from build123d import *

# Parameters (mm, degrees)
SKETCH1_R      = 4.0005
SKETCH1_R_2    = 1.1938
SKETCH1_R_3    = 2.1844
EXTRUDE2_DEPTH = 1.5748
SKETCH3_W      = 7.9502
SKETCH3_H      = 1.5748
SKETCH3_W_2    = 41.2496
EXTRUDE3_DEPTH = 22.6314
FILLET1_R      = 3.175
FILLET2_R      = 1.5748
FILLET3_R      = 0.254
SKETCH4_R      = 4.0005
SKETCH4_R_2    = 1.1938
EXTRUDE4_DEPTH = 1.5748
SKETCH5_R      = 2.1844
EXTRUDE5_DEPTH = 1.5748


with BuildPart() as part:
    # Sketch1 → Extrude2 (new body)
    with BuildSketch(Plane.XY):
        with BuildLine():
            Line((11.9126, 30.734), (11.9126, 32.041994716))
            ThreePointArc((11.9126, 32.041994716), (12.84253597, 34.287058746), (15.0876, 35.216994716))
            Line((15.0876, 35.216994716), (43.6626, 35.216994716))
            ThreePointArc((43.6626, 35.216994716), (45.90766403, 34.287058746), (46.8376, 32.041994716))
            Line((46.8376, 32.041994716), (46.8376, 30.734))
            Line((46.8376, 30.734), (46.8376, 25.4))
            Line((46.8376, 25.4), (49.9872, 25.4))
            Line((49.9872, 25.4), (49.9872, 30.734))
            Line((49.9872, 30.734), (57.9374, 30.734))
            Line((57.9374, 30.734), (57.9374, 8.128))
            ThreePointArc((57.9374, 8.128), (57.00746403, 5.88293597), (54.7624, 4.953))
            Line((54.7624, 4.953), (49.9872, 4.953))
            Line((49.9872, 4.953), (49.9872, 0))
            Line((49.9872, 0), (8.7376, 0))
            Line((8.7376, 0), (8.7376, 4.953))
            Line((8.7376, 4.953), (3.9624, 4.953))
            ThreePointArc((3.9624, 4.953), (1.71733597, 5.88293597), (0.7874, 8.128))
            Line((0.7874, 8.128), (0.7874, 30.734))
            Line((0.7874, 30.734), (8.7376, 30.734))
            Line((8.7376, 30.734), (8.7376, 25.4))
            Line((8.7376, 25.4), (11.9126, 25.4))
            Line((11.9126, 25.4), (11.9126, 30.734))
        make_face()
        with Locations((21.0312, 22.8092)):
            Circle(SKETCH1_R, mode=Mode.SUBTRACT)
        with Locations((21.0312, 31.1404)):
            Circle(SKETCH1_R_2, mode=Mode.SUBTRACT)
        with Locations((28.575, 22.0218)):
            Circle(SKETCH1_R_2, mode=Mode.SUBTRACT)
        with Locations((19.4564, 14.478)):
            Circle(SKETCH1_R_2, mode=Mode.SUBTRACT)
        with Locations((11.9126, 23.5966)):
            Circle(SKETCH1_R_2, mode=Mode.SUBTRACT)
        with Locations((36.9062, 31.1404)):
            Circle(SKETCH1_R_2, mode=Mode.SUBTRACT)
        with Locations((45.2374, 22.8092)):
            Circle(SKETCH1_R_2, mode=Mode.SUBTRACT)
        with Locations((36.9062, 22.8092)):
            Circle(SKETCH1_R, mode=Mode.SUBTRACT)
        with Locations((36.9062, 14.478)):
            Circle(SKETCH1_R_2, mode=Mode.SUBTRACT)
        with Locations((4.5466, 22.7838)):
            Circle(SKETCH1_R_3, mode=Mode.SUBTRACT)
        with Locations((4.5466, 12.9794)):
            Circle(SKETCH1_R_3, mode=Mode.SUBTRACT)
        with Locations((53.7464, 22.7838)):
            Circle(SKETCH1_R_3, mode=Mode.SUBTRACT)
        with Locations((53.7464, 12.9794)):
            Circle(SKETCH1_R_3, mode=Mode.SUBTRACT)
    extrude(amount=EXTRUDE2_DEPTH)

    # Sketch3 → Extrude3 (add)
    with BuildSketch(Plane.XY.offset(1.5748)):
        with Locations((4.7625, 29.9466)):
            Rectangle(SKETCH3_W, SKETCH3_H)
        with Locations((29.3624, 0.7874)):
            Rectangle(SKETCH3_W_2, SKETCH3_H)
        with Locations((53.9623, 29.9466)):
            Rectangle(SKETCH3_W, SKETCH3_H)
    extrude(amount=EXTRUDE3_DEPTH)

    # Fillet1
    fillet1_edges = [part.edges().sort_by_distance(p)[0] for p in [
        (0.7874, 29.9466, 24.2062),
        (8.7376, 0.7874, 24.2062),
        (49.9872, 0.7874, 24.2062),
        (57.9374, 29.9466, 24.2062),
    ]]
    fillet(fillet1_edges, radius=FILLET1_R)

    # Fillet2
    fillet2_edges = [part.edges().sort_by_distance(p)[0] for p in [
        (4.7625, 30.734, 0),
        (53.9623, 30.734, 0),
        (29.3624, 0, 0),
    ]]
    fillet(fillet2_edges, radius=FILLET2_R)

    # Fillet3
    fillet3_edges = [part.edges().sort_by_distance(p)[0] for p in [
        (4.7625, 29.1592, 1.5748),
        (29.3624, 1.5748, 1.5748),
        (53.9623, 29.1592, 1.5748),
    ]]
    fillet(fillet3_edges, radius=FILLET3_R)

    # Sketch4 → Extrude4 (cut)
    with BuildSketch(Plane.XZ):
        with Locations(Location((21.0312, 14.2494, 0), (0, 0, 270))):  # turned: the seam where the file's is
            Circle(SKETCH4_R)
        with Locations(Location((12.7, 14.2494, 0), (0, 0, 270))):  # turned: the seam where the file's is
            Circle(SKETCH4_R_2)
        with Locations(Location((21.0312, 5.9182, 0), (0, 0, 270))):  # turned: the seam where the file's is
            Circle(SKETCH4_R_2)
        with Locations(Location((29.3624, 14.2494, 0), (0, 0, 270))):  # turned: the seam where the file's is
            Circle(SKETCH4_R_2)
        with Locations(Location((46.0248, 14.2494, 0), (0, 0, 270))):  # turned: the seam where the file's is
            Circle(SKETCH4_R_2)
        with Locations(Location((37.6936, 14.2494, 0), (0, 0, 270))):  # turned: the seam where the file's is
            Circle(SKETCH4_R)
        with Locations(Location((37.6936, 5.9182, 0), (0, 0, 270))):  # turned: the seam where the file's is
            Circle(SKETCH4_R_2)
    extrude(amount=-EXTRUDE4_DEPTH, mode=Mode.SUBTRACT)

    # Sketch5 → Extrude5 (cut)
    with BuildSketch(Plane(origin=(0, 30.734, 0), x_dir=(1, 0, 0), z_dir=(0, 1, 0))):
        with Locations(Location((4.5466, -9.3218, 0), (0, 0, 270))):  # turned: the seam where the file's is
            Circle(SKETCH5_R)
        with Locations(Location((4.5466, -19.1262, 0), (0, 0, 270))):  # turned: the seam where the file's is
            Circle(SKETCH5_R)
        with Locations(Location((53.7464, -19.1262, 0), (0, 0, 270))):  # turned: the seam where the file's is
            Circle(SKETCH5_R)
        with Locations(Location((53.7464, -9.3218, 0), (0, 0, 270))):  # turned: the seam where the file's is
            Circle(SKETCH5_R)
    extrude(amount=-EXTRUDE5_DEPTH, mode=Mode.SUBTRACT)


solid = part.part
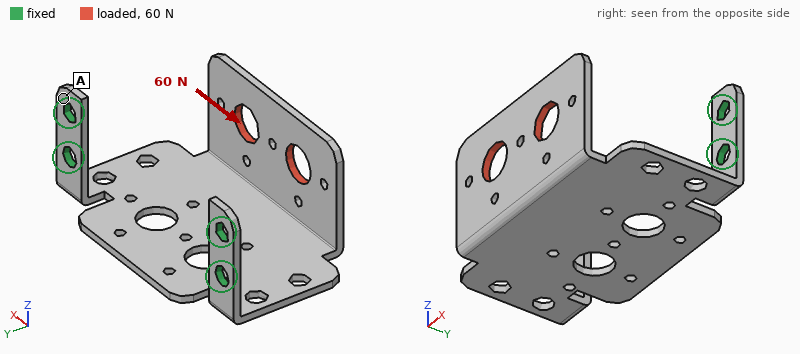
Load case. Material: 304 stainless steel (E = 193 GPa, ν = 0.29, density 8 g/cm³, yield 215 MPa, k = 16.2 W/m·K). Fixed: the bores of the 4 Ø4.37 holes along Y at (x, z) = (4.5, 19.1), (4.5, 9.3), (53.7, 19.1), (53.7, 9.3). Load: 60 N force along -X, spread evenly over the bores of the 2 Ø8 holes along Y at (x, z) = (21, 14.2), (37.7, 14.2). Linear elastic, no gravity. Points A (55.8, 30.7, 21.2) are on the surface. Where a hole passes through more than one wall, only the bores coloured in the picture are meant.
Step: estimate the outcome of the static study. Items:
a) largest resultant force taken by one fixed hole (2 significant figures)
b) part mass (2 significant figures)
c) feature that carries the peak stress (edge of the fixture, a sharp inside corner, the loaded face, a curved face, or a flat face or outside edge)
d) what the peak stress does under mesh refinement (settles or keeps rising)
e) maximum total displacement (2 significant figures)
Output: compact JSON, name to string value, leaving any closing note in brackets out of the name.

{"largest resultant force taken by one fixed hole": "49 N", "part mass": "34 g", "feature that carries the peak stress": "edge of the fixture", "what the peak stress does under mesh refinement": "keeps rising", "maximum total displacement": "0.13 mm"}
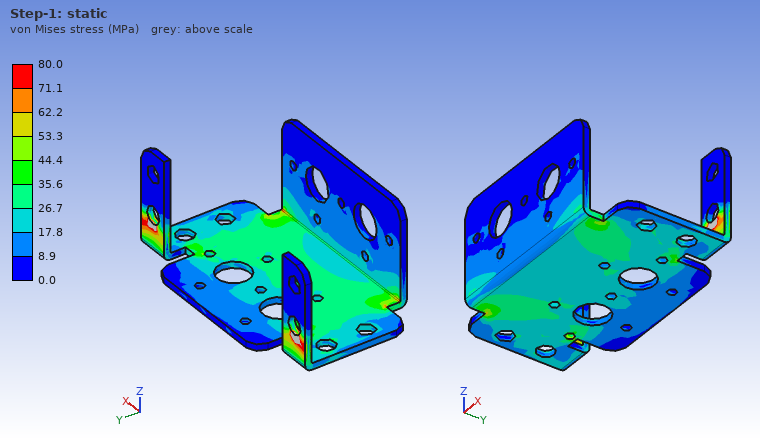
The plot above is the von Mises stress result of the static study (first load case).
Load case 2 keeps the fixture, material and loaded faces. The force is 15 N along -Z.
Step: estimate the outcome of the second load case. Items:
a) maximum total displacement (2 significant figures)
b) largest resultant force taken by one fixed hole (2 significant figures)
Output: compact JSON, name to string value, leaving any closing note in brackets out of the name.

{"maximum total displacement": "0.26 mm", "largest resultant force taken by one fixed hole": "7.4 N"}
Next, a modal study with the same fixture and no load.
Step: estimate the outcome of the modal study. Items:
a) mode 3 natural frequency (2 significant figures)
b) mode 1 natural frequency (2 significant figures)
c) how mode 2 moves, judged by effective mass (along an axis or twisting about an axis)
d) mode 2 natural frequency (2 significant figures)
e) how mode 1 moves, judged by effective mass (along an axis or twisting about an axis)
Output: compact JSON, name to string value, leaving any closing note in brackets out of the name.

{"mode 3 natural frequency": "1400 Hz", "mode 1 natural frequency": "330 Hz", "how mode 2 moves, judged by effective mass": "along X", "mode 2 natural frequency": "1000 Hz", "how mode 1 moves, judged by effective mass": "along Z"}
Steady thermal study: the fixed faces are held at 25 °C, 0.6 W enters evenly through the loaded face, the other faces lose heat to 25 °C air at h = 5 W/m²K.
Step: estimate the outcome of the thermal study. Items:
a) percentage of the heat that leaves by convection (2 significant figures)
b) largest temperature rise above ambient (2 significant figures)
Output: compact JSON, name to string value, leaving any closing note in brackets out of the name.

{"percentage of the heat that leaves by convection": "66 %", "largest temperature rise above ambient": "25 K"}
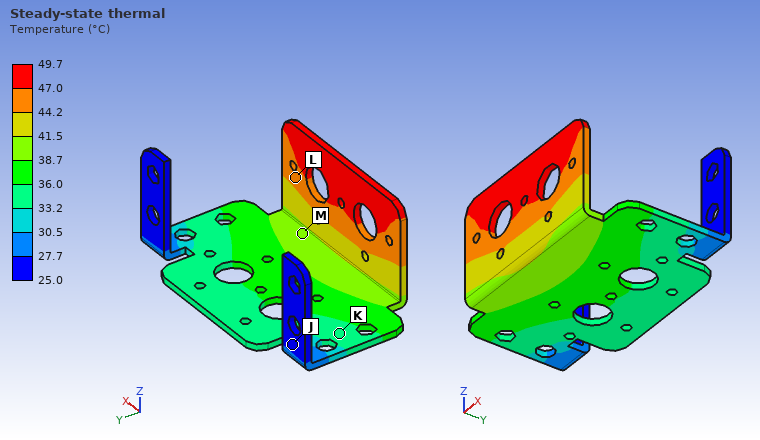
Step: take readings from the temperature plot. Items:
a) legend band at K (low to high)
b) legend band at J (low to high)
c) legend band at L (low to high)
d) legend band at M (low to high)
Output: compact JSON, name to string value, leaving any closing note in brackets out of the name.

{"legend band at K": "33.2 to 36.0 °C", "legend band at J": "25.0 to 27.7 °C", "legend band at L": "44.2 to 47.0 °C", "legend band at M": "38.7 to 41.5 °C"}
